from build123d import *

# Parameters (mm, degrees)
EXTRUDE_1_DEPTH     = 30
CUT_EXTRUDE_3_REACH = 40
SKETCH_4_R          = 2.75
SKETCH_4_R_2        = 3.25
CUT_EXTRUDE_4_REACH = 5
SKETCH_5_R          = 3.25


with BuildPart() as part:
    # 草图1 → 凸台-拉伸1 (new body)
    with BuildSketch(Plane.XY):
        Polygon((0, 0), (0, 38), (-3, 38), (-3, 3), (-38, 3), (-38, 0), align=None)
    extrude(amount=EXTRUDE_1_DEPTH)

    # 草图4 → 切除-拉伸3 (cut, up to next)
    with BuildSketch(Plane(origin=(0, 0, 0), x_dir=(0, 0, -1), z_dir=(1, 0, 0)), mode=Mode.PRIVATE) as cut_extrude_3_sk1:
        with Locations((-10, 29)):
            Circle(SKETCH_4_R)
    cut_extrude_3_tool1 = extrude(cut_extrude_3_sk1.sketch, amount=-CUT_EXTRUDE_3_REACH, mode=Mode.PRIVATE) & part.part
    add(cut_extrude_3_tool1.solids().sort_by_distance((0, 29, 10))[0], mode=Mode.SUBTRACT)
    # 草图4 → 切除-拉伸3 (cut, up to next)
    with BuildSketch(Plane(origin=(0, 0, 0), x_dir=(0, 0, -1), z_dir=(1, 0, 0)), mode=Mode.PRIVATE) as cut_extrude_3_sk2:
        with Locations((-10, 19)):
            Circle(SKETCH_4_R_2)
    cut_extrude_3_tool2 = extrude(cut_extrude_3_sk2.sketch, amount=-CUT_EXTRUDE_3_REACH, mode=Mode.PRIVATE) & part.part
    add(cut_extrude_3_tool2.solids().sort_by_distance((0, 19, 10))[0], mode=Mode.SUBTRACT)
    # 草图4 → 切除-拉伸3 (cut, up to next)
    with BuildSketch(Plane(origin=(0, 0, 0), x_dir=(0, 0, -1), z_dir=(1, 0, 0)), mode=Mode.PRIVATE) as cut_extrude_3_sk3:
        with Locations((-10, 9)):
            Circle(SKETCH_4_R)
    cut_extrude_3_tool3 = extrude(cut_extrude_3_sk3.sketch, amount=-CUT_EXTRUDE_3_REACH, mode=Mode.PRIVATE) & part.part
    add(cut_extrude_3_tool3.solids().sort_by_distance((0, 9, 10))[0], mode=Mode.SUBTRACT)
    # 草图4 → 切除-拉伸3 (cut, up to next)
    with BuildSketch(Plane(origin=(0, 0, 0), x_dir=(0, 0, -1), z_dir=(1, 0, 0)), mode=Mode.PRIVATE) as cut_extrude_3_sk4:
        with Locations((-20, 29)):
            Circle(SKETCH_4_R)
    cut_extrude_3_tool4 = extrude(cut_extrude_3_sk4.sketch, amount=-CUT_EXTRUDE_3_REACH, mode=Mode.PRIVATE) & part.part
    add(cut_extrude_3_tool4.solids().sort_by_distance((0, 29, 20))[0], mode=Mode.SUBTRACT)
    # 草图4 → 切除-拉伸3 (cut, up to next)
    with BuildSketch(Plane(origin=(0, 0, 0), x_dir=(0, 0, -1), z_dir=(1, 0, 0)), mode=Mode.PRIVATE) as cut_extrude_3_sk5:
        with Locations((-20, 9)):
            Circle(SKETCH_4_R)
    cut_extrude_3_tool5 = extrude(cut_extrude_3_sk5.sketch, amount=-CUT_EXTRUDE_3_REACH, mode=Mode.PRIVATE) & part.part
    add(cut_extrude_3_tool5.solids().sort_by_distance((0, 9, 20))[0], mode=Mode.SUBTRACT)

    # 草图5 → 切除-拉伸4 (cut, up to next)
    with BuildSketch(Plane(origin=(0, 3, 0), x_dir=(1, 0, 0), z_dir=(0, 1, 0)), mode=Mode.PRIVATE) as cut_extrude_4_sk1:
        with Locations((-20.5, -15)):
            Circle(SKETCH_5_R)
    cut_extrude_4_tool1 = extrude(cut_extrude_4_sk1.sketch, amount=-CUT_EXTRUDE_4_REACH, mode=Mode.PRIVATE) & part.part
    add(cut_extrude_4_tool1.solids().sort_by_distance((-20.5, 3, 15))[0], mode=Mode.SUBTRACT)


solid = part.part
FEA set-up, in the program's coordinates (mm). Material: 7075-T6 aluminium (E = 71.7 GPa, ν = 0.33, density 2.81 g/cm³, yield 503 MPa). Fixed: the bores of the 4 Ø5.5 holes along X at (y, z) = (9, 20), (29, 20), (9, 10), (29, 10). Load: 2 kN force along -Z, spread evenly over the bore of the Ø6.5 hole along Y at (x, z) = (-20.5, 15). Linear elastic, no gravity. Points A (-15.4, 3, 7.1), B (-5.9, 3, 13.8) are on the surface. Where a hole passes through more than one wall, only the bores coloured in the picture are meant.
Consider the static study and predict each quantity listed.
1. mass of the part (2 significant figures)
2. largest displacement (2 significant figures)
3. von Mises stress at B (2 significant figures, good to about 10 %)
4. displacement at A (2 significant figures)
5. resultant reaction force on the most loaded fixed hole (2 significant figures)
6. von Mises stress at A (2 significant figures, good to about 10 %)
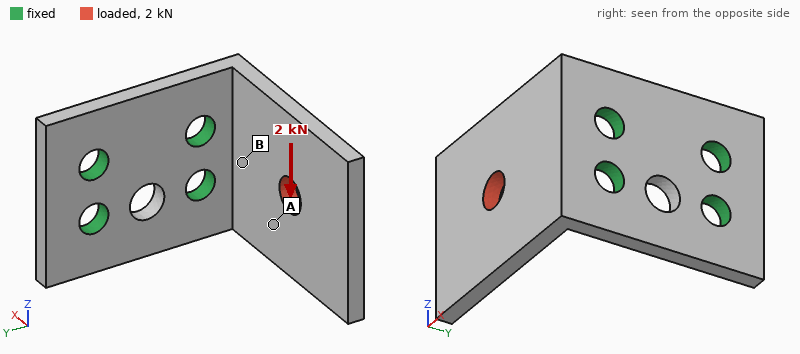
17 g
0.41 mm
180 MPa
0.17 mm
2.8 kN
74 MPa
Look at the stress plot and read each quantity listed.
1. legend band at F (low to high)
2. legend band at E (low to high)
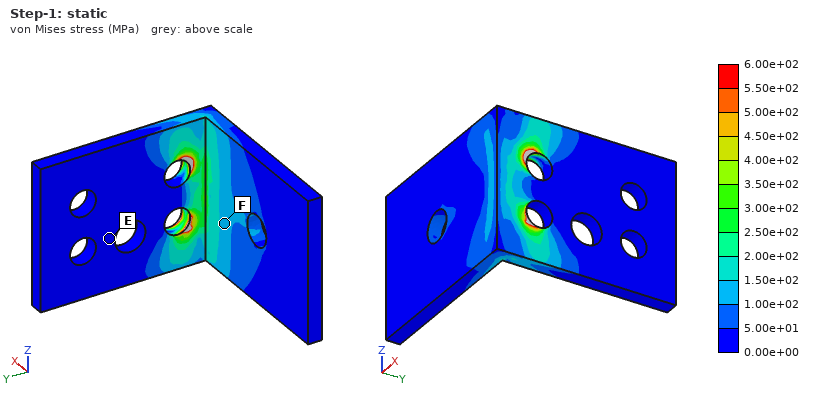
1.00e+02 to 1.50e+02 MPa
0.00e+00 to 5.00e+01 MPa
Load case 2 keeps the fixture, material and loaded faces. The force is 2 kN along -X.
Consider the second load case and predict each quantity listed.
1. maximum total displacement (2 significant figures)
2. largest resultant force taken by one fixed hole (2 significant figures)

0.27 mm
1.0 kN
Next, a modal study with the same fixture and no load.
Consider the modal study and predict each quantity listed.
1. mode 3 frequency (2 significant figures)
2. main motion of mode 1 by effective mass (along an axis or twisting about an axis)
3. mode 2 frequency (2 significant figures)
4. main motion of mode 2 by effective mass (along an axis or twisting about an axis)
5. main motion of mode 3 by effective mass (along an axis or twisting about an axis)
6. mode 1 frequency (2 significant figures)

5300 Hz
along Y
4100 Hz
along Z
along Z
1500 Hz
